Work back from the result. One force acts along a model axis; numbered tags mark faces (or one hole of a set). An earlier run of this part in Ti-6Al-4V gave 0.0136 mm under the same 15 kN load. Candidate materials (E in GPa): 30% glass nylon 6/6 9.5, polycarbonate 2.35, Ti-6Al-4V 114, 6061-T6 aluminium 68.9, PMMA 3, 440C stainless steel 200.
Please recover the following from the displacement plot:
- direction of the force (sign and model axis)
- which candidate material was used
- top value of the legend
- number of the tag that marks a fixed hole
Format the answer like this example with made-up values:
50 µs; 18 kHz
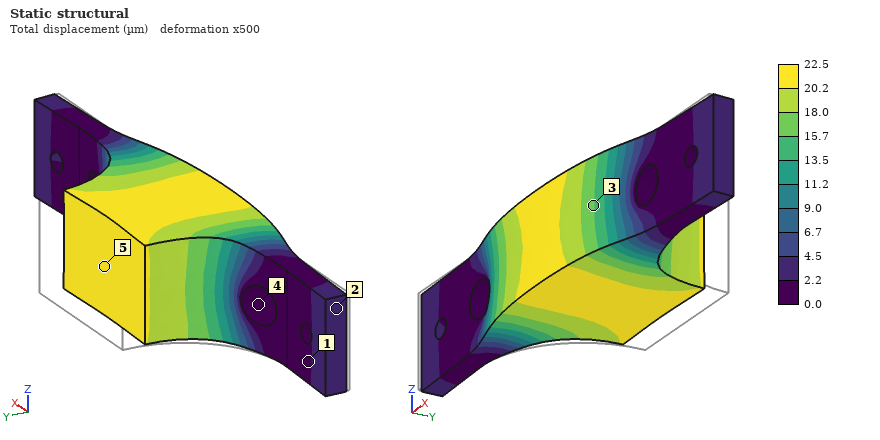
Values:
-Y; 6061-T6 aluminium; 22.5 µm; 4
